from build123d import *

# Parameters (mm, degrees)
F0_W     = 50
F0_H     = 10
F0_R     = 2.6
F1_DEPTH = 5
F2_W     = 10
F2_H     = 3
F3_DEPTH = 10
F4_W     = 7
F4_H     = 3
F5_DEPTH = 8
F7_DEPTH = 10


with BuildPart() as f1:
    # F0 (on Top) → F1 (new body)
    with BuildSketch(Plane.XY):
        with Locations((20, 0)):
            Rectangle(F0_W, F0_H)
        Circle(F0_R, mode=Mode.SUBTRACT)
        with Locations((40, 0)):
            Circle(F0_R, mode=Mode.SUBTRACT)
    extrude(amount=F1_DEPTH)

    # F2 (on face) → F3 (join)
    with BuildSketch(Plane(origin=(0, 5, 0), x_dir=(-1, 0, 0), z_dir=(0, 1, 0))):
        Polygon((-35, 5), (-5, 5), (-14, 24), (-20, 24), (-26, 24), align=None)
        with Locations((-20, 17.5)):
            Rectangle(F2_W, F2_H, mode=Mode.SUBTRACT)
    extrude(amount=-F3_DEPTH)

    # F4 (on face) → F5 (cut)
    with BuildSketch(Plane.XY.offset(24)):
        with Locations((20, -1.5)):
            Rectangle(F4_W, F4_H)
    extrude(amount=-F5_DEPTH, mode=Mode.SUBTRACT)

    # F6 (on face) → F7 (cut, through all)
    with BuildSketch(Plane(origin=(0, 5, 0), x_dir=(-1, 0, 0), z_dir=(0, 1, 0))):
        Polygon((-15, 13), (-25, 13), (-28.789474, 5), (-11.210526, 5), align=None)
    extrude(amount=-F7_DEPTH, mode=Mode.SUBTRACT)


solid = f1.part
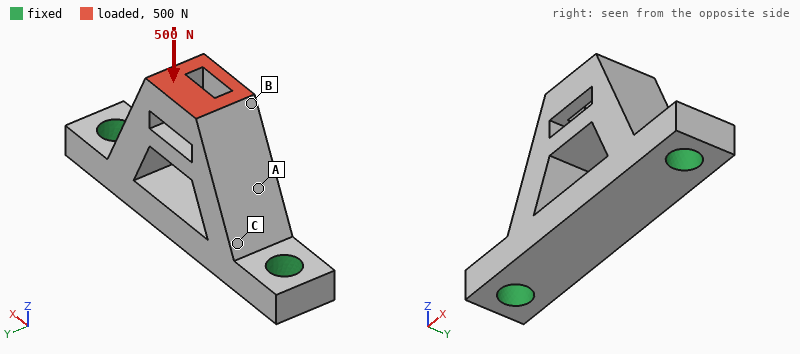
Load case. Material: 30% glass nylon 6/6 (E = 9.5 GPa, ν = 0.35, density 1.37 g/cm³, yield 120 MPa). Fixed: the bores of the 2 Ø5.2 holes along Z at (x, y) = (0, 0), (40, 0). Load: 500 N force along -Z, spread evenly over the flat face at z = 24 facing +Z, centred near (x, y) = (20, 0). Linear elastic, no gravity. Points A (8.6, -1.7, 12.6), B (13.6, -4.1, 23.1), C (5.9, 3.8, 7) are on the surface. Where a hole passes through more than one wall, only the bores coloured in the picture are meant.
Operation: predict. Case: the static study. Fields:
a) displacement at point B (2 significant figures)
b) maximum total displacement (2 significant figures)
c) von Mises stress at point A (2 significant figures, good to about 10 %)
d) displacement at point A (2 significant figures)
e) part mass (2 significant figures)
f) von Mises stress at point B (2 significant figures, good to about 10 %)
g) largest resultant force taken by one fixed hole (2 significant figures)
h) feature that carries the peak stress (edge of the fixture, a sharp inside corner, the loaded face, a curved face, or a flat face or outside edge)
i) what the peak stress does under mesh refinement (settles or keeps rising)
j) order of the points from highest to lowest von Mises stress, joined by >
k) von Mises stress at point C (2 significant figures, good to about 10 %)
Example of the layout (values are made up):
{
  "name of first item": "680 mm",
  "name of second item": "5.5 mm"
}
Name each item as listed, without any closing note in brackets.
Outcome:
{
  "displacement at point B": "25 µm",
  "maximum total displacement": "44 µm",
  "von Mises stress at point A": "7.5 MPa",
  "displacement at point A": "19 µm",
  "part mass": "6.5 g",
  "von Mises stress at point B": "3.5 MPa",
  "largest resultant force taken by one fixed hole": "280 N",
  "feature that carries the peak stress": "edge of the fixture",
  "what the peak stress does under mesh refinement": "keeps rising",
  "order of the points from highest to lowest von Mises stress, joined by >": "C > A > B",
  "von Mises stress at point C": "12 MPa"
}
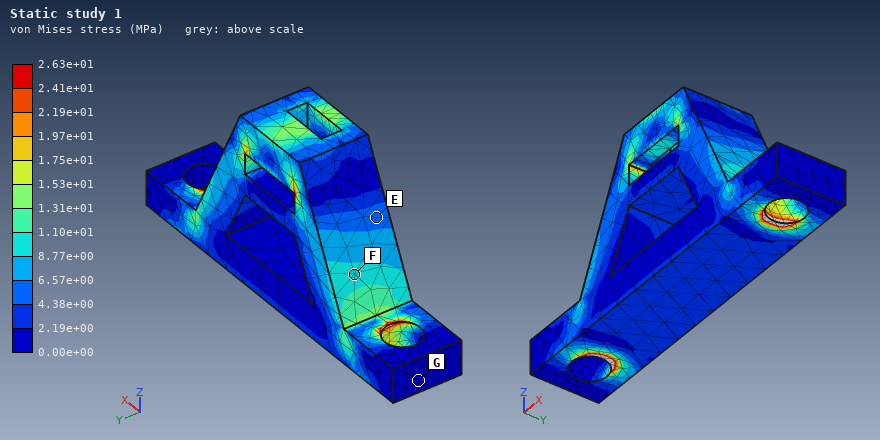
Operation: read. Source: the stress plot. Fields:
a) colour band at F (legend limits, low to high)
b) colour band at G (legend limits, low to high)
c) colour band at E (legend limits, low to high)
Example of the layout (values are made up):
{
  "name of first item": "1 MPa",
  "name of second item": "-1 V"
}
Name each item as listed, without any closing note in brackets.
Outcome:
{
  "colour band at F": "8.77e+00 to 1.10e+01 MPa",
  "colour band at G": "0.00e+00 to 2.19e+00 MPa",
  "colour band at E": "4.38e+00 to 6.57e+00 MPa"
}
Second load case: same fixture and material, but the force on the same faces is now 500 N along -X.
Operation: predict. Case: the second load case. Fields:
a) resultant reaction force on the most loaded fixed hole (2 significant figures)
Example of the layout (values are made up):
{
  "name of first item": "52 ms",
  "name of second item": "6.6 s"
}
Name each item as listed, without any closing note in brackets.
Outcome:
{
  "resultant reaction force on the most loaded fixed hole": "410 N"
}
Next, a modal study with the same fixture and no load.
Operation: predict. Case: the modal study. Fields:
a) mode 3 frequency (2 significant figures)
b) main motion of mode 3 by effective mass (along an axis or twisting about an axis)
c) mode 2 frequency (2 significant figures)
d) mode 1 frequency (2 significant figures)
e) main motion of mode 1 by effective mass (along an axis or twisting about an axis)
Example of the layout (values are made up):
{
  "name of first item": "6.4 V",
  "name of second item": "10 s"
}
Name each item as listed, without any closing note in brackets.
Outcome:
{
  "mode 3 frequency": "10 kHz",
  "main motion of mode 3 by effective mass": "along Z",
  "mode 2 frequency": "9700 Hz",
  "mode 1 frequency": "3800 Hz",
  "main motion of mode 1 by effective mass": "along Y"
}
